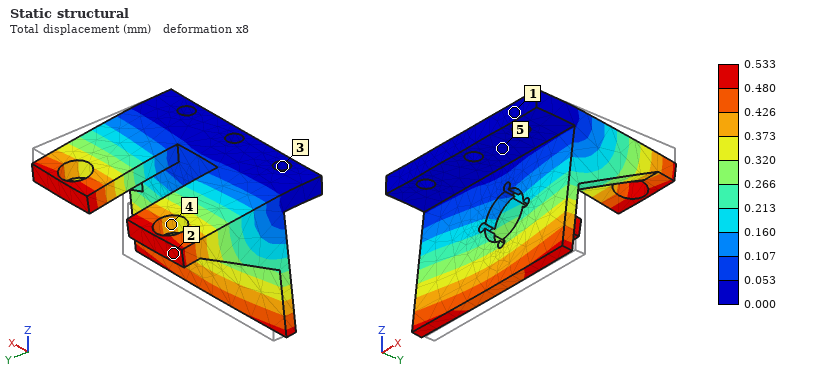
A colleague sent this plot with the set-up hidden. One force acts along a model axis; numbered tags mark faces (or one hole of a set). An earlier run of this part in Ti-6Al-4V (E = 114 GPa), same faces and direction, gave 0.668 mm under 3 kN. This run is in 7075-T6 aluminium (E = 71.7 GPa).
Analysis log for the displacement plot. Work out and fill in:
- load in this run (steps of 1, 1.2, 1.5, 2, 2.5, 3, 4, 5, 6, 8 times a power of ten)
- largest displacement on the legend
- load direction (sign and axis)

1.5 kN
0.533 mm
-Z
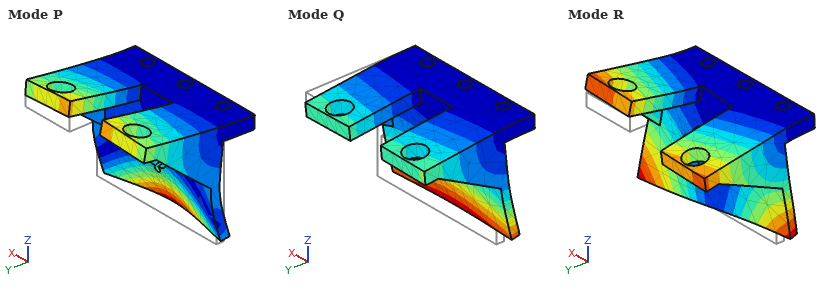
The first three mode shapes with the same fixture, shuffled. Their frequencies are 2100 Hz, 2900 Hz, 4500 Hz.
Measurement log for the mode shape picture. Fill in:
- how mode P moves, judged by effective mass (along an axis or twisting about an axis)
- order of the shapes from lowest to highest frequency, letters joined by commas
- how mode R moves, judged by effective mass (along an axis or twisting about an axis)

along Z
Q, R, P
twisting about Y
